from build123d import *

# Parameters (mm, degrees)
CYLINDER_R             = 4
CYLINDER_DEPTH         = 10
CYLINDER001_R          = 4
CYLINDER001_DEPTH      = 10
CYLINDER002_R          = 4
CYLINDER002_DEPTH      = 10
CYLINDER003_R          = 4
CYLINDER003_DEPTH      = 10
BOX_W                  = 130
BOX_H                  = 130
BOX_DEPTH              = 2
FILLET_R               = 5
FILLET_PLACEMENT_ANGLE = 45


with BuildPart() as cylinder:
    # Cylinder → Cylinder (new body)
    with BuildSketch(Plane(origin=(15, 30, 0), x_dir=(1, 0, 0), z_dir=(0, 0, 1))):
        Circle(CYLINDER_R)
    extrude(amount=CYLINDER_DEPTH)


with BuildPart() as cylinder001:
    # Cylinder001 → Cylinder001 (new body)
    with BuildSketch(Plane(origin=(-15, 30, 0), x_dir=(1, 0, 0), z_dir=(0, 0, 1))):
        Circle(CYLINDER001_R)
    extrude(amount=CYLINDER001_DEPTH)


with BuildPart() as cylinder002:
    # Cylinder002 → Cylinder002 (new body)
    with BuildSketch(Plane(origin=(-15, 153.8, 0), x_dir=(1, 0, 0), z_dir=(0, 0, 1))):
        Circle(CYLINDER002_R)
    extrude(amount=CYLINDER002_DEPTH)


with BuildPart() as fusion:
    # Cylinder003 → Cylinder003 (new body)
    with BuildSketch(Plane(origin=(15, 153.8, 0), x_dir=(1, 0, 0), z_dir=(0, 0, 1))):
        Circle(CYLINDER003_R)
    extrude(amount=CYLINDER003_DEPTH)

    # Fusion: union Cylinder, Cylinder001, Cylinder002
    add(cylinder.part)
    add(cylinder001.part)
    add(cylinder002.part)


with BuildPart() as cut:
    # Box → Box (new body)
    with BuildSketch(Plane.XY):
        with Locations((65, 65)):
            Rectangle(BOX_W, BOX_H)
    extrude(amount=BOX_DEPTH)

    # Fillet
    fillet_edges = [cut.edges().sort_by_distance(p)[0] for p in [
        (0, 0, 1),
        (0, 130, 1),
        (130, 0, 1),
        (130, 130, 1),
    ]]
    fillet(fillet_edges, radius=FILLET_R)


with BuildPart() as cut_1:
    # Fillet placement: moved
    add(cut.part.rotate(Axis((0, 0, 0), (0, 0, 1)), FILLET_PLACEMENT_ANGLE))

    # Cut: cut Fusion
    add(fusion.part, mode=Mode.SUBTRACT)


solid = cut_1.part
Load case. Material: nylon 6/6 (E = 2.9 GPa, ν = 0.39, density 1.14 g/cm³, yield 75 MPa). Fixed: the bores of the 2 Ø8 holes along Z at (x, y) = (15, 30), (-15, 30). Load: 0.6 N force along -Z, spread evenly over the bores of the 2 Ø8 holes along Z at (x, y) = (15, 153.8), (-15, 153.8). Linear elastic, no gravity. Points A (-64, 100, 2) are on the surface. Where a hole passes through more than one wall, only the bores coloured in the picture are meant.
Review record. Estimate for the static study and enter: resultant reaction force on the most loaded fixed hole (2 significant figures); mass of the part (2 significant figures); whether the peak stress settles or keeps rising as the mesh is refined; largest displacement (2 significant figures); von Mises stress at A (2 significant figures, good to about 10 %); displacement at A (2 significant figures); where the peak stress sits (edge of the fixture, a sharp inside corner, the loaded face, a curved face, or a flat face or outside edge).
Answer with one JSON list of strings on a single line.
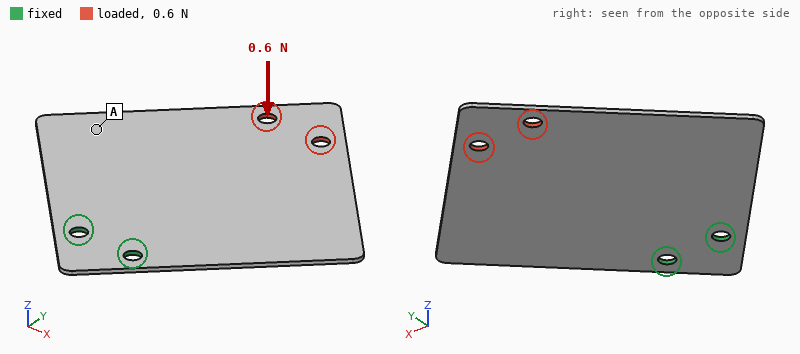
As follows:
["0.30 N", "38 g", "keeps rising", "2.4 mm", "0.23 MPa", "0.69 mm", "edge of the fixture"]
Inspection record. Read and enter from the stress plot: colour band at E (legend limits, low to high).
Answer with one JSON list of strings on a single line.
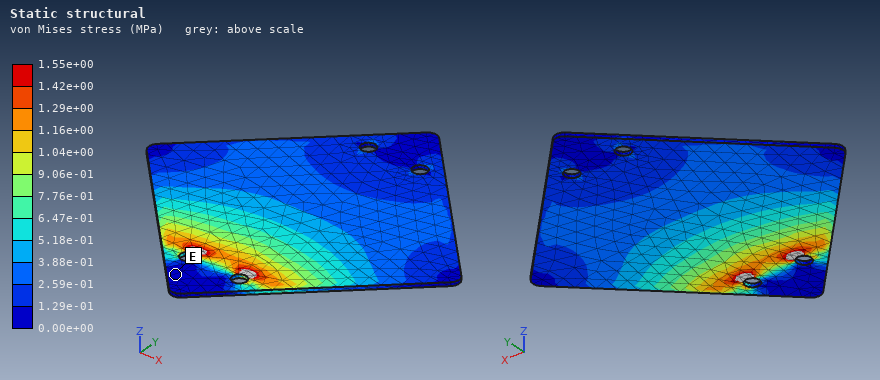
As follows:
["0.00e+00 to 1.29e-01 MPa"]
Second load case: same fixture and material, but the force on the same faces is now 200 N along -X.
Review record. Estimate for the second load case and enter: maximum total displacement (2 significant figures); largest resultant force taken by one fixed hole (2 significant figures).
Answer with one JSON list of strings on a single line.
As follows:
["1.4 mm", "690 N"]
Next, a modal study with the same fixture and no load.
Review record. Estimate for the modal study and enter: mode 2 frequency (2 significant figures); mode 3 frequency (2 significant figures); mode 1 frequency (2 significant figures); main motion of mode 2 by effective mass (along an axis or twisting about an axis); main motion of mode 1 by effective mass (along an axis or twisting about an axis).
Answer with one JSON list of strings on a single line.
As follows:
["58 Hz", "120 Hz", "29 Hz", "twisting about Y", "along Z"]
